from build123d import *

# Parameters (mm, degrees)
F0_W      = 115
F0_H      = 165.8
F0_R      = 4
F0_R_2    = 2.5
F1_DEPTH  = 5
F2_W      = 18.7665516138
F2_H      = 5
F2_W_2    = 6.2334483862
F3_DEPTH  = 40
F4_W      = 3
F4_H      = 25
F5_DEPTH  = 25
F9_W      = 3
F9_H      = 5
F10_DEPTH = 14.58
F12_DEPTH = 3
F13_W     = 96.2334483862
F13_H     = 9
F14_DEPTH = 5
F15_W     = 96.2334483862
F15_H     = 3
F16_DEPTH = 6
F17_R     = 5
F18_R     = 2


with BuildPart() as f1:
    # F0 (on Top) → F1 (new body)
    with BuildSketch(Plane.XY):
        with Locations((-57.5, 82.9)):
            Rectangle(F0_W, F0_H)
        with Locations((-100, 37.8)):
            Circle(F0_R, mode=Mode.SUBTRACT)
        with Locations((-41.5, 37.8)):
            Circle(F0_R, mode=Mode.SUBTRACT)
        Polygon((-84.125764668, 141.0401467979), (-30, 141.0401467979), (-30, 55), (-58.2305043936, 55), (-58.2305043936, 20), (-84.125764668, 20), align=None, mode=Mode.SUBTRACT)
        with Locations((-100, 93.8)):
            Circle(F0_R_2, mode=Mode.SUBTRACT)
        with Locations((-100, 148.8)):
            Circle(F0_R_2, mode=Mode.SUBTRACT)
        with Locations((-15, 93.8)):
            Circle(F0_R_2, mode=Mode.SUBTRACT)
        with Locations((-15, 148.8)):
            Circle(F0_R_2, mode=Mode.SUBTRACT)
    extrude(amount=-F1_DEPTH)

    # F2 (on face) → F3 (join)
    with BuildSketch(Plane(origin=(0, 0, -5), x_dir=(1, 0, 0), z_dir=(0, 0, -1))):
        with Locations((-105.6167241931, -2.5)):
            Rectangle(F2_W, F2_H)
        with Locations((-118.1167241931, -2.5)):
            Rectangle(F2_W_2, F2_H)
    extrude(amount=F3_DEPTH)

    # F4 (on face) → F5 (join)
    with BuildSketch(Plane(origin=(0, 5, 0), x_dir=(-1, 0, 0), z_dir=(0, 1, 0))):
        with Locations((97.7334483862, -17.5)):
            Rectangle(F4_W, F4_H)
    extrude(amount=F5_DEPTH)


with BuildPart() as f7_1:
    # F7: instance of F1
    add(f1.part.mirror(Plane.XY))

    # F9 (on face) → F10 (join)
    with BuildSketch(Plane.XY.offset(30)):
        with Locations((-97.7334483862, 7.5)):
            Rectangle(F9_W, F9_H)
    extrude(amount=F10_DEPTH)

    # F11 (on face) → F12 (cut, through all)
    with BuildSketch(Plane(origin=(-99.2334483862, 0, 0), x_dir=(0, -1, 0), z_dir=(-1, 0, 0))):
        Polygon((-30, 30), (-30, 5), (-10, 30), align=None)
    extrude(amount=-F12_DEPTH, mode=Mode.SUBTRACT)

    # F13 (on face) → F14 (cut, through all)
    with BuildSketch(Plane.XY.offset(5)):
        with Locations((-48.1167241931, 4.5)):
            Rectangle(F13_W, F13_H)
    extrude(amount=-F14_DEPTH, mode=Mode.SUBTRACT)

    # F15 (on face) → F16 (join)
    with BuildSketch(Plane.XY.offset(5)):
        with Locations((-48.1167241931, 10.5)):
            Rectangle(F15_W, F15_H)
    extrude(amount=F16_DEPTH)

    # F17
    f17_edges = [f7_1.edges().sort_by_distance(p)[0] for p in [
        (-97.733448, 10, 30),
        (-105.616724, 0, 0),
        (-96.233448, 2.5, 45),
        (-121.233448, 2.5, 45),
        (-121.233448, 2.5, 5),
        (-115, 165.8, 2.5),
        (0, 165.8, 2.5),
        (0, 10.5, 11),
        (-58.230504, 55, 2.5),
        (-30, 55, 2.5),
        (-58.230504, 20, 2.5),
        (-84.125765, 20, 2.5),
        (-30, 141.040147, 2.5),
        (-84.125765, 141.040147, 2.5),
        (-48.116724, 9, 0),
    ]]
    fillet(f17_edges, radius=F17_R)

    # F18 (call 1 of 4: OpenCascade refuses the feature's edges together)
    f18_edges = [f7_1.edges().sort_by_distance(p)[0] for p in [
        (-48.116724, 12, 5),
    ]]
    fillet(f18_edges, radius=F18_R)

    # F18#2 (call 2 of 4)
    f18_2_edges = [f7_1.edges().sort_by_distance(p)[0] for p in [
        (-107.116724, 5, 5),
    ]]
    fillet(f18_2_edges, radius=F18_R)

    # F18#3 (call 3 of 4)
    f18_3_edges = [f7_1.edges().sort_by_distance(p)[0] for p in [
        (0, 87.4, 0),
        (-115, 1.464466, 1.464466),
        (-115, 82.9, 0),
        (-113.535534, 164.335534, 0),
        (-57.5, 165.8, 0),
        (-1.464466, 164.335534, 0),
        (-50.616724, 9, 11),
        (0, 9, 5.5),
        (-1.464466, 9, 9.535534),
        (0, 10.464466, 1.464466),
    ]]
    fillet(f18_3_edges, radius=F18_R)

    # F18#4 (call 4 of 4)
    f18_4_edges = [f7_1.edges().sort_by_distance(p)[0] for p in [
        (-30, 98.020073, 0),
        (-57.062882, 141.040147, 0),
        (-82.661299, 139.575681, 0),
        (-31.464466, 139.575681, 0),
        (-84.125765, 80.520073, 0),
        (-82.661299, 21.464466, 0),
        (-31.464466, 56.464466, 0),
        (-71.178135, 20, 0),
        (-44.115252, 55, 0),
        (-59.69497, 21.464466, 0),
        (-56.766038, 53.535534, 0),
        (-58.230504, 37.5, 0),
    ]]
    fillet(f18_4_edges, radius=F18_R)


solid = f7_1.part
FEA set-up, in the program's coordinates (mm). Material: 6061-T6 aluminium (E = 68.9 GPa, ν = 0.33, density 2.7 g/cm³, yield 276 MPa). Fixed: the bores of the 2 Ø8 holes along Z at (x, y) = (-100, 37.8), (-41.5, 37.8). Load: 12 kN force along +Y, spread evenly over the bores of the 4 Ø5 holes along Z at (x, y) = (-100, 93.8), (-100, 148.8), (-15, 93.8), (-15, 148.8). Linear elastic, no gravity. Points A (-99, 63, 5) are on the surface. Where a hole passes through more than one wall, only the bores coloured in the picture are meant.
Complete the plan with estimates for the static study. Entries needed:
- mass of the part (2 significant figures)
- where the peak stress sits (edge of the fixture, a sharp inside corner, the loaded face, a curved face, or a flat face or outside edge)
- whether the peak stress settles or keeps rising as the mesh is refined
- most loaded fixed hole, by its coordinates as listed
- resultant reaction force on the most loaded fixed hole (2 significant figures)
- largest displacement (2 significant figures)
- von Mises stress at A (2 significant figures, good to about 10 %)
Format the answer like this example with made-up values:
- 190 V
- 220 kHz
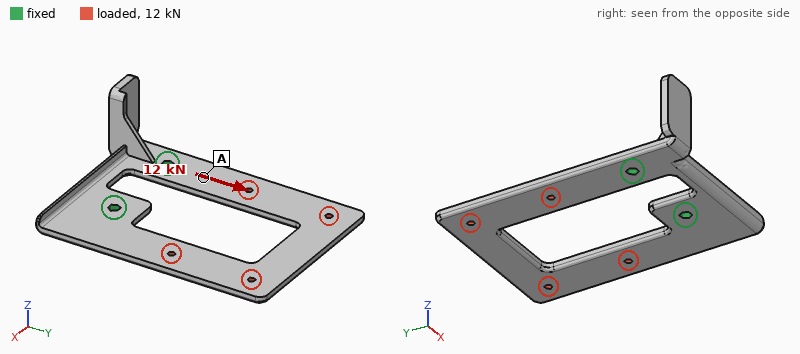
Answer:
- 190 g
- edge of the fixture
- keeps rising
- (-41.5, 37.8)
- 7.1 kN
- 0.25 mm
- 42 MPa
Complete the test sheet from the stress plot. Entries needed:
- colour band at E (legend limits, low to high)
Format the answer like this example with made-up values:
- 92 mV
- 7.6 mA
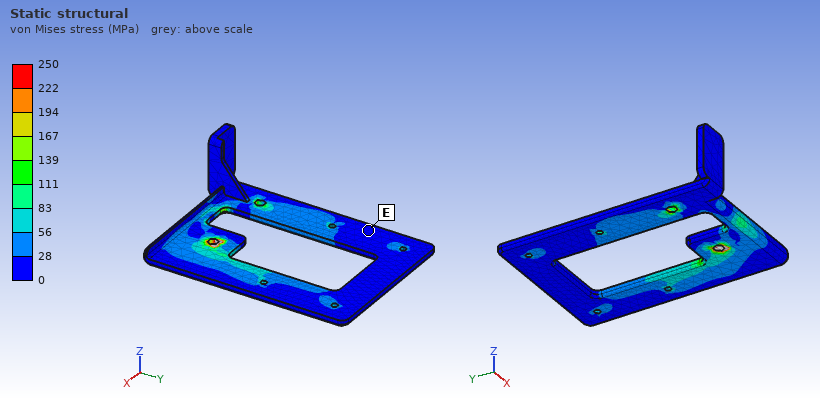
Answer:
- 0 to 28 MPa
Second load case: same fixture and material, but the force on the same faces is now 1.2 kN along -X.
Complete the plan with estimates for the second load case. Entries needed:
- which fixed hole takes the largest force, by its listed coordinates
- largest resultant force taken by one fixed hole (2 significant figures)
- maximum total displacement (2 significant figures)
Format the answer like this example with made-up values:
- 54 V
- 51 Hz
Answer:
- (-41.5, 37.8)
- 1.2 kN
- 0.20 mm
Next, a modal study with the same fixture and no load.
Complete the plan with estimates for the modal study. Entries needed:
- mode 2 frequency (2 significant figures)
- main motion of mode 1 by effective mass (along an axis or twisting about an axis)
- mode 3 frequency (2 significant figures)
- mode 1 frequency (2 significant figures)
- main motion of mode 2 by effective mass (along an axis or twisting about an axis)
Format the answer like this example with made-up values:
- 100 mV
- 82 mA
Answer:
- 490 Hz
- along Z
- 1300 Hz
- 200 Hz
- twisting about Y
